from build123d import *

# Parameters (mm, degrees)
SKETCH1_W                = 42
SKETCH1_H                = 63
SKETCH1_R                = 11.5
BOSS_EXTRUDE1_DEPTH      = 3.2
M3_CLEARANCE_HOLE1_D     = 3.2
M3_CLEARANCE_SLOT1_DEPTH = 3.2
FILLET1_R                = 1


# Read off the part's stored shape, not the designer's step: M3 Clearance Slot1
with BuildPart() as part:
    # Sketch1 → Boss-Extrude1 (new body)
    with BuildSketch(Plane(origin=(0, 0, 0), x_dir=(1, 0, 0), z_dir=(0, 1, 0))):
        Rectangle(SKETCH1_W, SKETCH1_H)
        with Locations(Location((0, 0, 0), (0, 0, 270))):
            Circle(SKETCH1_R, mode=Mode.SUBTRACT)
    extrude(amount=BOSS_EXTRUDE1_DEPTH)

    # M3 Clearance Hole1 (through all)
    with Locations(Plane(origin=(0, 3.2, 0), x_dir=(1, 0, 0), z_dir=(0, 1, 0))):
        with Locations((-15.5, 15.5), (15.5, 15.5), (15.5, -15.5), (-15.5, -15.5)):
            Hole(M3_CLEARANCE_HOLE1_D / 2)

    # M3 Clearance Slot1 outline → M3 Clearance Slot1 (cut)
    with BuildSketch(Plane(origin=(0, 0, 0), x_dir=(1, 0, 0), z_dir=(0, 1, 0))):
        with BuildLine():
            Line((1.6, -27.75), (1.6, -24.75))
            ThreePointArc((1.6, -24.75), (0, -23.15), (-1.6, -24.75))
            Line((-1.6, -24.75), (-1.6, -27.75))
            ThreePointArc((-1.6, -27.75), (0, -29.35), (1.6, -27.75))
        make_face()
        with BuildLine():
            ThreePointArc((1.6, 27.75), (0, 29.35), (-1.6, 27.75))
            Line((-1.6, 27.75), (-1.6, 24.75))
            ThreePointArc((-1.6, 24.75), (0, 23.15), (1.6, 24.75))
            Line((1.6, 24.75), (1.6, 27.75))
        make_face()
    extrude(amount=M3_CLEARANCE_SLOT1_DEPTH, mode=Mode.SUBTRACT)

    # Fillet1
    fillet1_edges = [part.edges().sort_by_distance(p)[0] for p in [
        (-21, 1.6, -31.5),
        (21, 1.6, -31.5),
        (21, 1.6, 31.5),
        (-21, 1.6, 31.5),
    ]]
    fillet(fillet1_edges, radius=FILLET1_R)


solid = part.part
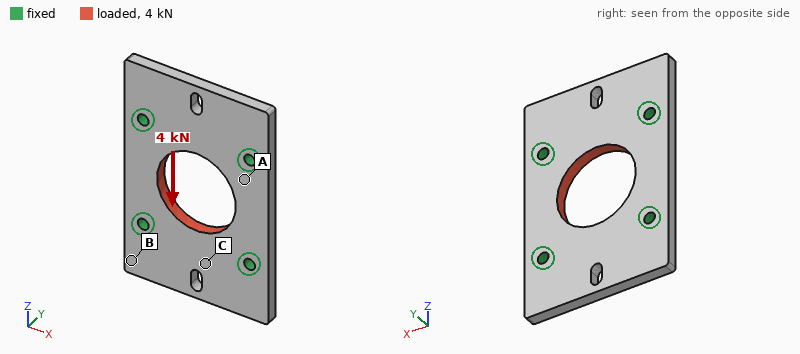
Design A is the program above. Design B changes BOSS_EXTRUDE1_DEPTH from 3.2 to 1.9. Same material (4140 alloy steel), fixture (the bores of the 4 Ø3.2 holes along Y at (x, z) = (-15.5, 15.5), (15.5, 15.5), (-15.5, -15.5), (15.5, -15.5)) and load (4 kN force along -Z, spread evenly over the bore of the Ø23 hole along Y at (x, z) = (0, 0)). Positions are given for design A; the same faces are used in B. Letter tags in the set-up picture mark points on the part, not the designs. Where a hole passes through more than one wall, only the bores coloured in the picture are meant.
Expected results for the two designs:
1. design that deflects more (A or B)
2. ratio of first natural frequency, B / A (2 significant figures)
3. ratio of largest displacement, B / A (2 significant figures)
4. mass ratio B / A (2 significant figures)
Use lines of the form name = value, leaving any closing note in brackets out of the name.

design that deflects more = B
ratio of first natural frequency, B / A = 0.63
ratio of largest displacement, B / A = 1.7
mass ratio B / A = 0.59
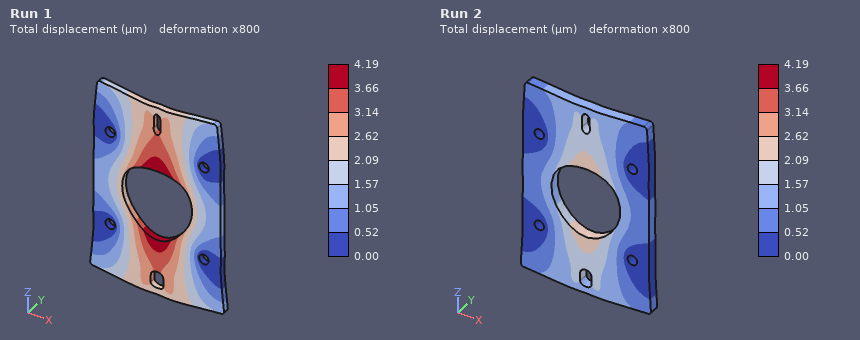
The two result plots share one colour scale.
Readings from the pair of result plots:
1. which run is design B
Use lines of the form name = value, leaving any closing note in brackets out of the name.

which run is design B = Run 1
